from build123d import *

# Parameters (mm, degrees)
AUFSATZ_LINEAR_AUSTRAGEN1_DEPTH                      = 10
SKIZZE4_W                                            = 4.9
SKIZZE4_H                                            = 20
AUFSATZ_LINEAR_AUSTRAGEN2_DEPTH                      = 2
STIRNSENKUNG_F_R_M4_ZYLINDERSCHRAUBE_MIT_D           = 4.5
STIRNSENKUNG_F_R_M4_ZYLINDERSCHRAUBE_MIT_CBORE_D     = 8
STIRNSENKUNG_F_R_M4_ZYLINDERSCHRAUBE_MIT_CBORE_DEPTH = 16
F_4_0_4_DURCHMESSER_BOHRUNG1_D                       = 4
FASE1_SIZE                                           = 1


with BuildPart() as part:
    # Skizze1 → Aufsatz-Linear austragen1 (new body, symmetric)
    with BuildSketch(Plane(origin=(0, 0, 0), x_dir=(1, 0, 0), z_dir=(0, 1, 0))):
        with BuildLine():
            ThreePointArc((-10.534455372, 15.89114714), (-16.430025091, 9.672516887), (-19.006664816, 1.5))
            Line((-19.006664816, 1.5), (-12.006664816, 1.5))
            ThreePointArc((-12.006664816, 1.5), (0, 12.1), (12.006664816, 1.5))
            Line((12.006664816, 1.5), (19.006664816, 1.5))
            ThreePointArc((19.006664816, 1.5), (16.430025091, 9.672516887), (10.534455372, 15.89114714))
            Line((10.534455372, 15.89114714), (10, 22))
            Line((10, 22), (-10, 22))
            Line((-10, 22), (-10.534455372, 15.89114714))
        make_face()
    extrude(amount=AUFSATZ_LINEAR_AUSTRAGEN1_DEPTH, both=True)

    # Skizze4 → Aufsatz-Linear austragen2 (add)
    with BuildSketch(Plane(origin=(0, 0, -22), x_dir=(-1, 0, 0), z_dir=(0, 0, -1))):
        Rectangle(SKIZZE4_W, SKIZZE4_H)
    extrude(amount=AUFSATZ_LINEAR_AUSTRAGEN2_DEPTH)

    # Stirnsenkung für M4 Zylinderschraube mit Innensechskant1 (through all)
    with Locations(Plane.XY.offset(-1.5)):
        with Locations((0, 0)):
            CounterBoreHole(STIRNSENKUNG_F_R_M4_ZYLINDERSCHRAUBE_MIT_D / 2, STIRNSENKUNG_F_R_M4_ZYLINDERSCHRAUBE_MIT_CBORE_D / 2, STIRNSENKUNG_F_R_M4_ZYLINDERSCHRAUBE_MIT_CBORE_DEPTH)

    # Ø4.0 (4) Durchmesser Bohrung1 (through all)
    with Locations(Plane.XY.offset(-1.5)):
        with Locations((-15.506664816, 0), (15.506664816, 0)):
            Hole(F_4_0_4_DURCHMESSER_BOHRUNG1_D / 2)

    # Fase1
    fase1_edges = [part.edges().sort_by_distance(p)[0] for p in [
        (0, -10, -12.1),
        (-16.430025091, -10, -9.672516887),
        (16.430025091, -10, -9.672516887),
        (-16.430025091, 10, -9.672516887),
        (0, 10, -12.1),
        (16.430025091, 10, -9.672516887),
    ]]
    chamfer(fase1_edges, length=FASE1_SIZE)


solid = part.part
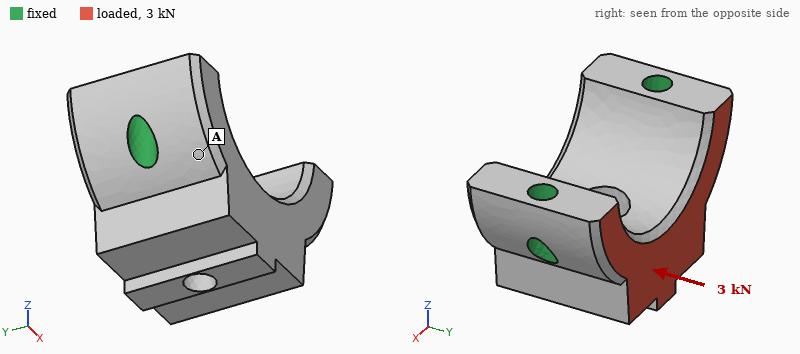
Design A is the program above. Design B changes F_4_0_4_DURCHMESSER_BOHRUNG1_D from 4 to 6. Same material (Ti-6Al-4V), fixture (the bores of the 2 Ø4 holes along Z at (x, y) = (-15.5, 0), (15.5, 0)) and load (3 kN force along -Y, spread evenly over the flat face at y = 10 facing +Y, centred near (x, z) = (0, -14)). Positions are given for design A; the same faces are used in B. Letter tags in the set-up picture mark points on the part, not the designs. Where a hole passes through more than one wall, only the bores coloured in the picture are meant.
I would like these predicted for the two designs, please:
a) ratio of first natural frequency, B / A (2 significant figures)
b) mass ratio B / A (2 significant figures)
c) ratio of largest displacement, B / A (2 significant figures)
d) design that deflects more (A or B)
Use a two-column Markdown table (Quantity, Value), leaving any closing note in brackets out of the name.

| Quantity | Value |
|---|---|
| ratio of first natural frequency, B / A | 1.2 |
| mass ratio B / A | 0.96 |
| ratio of largest displacement, B / A | 0.70 |
| design that deflects more | A |
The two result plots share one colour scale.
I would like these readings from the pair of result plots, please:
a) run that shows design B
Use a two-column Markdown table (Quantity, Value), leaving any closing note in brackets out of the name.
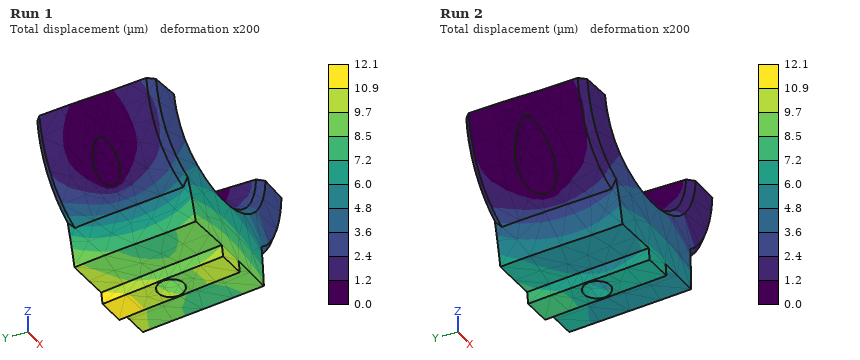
| Quantity | Value |
|---|---|
| run that shows design B | Run 2 |
